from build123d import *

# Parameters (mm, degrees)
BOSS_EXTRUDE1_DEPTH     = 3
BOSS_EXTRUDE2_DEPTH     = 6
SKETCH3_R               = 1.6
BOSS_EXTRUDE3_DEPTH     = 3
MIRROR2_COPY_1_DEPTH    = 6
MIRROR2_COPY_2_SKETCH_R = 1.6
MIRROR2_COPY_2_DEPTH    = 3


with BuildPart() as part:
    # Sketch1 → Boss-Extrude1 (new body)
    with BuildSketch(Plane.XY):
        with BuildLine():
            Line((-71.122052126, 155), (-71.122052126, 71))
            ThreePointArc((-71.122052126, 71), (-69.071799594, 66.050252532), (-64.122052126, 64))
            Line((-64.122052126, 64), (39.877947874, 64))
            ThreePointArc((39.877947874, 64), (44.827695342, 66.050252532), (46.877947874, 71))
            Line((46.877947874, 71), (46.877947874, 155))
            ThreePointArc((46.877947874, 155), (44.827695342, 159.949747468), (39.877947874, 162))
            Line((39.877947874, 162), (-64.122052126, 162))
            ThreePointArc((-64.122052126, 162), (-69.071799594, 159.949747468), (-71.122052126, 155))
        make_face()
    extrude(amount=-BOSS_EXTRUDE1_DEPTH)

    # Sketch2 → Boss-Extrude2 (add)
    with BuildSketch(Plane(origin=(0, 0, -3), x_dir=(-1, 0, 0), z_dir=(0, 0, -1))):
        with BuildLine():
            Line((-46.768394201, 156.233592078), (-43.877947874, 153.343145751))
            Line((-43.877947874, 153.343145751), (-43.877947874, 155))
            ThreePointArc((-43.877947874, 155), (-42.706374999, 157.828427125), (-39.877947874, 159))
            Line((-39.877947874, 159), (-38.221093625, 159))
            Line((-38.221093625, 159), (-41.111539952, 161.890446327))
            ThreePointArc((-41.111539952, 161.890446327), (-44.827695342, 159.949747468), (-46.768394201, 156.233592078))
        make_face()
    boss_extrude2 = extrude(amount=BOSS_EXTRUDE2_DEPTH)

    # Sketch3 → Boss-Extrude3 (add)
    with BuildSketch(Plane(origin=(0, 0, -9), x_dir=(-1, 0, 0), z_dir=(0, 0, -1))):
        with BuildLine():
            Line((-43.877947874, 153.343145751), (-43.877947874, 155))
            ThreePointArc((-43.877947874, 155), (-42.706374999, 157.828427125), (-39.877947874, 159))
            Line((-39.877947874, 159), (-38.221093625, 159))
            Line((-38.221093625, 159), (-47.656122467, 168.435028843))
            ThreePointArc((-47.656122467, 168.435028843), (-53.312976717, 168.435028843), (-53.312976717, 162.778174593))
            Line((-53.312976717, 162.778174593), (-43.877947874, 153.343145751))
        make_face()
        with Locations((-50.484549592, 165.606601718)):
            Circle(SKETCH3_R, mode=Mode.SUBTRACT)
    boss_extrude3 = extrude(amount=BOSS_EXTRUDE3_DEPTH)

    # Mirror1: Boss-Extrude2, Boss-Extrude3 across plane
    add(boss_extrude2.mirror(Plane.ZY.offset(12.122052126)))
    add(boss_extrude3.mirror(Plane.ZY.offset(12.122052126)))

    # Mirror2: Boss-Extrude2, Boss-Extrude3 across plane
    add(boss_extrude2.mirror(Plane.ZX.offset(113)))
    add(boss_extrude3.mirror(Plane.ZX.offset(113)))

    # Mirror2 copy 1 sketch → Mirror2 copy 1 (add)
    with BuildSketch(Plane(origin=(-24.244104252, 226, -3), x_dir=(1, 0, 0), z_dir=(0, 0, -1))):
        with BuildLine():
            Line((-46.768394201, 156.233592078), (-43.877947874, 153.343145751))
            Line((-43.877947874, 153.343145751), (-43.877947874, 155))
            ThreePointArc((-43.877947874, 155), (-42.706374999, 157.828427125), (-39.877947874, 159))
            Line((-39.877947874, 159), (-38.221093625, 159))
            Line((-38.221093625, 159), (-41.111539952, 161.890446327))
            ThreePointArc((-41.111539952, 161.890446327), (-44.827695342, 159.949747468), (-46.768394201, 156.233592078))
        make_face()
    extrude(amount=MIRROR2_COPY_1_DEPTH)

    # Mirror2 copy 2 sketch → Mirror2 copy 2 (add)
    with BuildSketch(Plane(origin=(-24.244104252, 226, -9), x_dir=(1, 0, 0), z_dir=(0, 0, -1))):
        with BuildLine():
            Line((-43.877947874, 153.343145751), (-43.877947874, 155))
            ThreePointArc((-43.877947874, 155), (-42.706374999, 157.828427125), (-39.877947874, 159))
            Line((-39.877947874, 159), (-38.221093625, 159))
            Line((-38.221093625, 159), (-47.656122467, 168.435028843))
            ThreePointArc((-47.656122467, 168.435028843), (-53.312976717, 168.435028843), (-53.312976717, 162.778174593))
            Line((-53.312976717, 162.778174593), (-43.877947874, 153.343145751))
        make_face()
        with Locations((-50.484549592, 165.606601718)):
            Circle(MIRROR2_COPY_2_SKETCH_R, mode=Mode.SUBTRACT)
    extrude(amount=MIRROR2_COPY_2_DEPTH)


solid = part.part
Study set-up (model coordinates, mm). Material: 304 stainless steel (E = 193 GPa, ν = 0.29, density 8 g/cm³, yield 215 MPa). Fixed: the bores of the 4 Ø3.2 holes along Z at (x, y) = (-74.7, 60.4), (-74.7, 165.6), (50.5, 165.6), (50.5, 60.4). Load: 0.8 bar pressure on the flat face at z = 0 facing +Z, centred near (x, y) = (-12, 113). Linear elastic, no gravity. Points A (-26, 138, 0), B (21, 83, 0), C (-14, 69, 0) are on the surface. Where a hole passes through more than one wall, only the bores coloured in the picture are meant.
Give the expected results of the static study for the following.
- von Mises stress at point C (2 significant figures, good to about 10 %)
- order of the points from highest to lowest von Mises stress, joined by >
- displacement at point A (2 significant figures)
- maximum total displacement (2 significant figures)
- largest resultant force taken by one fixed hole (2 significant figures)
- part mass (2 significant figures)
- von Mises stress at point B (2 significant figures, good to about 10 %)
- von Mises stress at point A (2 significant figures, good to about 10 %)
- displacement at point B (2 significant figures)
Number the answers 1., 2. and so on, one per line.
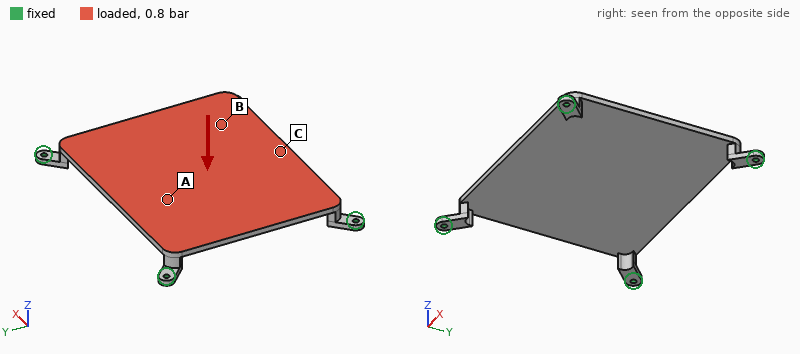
1. 49 MPa
2. C > A > B
3. 0.17 mm
4. 0.20 mm
5. 550 N
6. 290 g
7. 24 MPa
8. 37 MPa
9. 0.11 mm
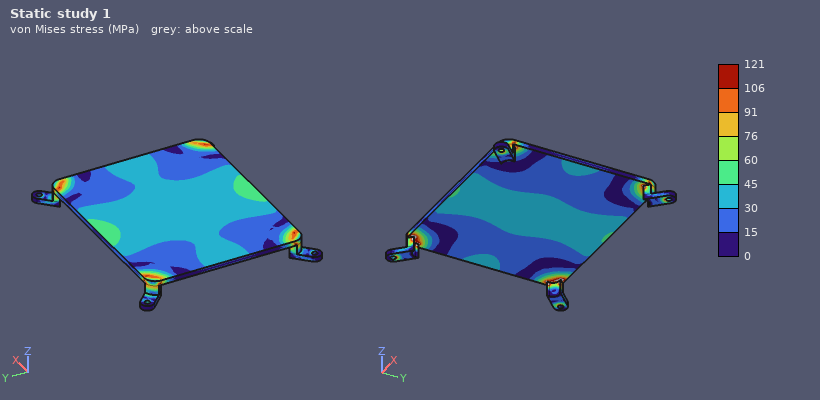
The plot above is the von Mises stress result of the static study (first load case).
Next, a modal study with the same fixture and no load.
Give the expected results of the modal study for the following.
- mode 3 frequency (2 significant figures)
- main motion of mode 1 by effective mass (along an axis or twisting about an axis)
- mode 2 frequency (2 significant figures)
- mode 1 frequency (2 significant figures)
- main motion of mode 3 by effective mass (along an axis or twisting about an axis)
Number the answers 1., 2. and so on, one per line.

1. 1400 Hz
2. along Z
3. 1300 Hz
4. 760 Hz
5. along X
